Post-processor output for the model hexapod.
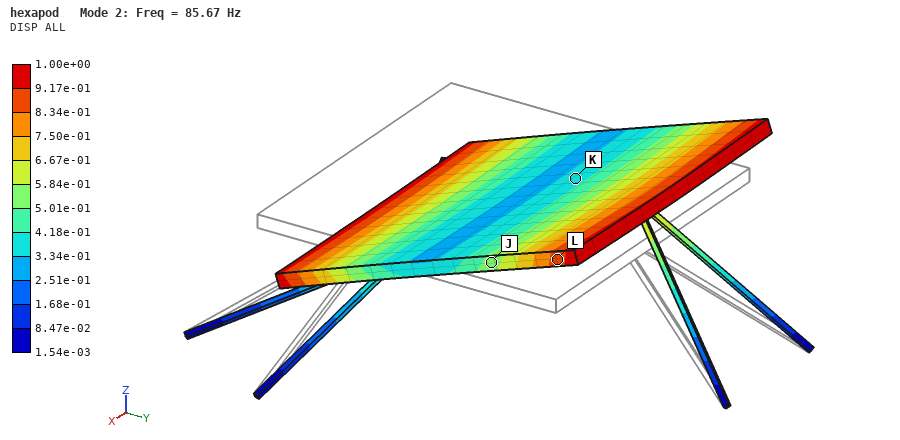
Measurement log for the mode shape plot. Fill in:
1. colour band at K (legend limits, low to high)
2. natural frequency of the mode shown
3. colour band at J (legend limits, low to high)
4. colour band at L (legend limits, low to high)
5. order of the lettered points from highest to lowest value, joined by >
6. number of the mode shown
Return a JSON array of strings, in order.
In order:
["3.34e-01 to 4.18e-01", "85.67 Hz", "5.01e-01 to 5.84e-01", "8.34e-01 to 9.17e-01", "L > J > K", "2"]
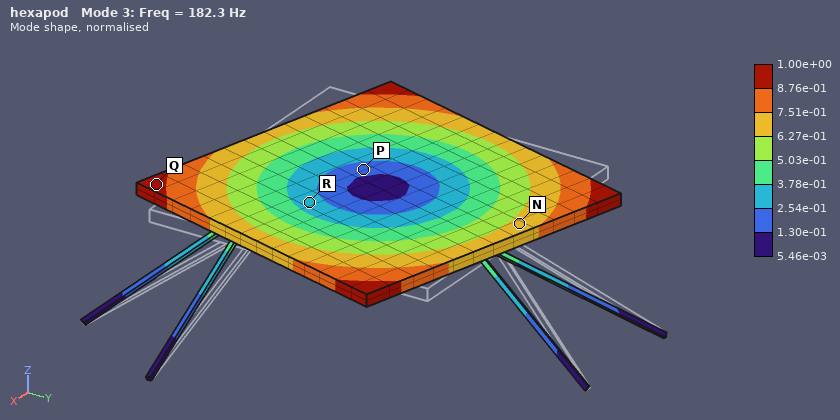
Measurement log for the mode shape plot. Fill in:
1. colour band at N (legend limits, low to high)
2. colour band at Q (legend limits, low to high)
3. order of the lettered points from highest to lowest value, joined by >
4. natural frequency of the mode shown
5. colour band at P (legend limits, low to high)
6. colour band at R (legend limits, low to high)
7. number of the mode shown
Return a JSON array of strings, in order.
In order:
["6.27e-01 to 7.51e-01", "8.76e-01 to 1.00e+00", "Q > N > R > P", "182.3 Hz", "1.30e-01 to 2.54e-01", "2.54e-01 to 3.78e-01", "3"]
